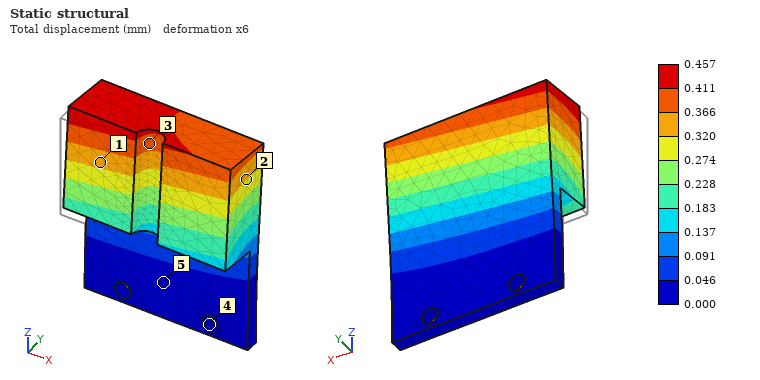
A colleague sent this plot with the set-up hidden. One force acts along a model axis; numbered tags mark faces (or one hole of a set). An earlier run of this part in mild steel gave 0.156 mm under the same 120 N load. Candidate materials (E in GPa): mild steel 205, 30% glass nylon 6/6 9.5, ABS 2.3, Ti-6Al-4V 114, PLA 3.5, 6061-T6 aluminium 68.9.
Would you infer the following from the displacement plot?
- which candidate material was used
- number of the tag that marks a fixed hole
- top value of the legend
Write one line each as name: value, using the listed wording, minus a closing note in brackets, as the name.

which candidate material was used: 6061-T6 aluminium
number of the tag that marks a fixed hole: 4
top value of the legend: 0.457 mm
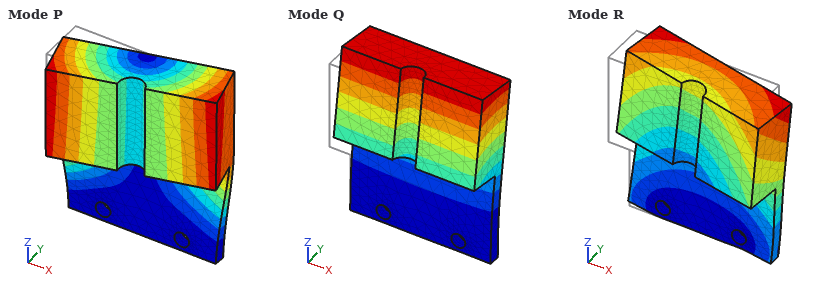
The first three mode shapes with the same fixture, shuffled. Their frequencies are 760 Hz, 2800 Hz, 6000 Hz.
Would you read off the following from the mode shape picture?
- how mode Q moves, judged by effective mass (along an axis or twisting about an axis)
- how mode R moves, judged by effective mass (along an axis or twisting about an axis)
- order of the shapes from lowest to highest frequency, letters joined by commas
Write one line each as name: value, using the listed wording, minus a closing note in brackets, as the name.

how mode Q moves, judged by effective mass: along Y
how mode R moves, judged by effective mass: along X
order of the shapes from lowest to highest frequency, letters joined by commas: Q, P, R
